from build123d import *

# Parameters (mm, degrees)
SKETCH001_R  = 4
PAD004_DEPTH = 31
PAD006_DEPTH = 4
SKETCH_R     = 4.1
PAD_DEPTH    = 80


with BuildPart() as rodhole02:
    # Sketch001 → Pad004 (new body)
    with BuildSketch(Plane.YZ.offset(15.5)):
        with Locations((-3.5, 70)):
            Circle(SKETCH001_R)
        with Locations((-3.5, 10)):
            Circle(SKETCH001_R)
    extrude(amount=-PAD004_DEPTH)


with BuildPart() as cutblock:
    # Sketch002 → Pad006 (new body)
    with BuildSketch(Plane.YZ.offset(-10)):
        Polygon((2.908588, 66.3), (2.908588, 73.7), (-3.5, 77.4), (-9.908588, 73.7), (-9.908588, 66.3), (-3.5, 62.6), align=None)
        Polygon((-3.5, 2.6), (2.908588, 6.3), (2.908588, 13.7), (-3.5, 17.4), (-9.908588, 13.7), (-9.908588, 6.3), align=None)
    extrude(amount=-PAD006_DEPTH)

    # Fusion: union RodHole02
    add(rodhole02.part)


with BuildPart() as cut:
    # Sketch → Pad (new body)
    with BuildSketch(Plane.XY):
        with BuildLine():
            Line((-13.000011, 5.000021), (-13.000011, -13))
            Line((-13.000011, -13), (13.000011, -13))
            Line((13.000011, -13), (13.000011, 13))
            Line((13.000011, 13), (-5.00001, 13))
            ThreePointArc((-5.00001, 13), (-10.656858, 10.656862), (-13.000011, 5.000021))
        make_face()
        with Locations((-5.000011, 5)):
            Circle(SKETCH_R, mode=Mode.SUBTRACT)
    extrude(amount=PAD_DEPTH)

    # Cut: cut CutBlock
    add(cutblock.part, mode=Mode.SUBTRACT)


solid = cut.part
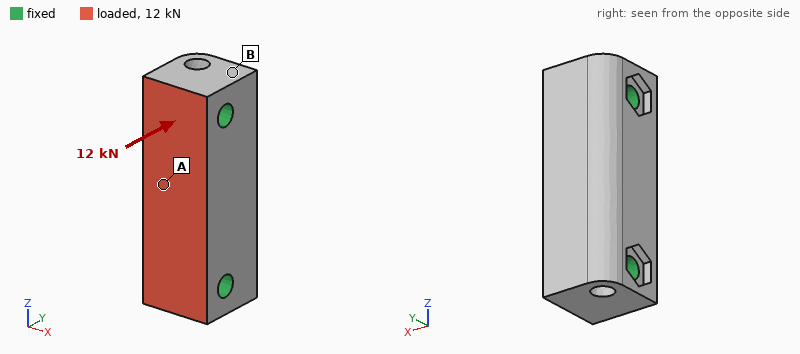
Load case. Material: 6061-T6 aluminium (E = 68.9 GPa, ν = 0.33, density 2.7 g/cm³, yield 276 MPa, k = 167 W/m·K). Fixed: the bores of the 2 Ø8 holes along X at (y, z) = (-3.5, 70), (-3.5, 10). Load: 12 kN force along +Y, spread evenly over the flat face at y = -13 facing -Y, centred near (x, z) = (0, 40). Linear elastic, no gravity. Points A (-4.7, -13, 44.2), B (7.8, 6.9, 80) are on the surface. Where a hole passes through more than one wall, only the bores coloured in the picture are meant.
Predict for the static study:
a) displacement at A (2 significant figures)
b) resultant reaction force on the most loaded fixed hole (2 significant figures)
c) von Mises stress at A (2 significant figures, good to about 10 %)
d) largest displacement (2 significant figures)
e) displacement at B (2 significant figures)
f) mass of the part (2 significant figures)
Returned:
9.6 µm
6.0 kN
12 MPa
11 µm
1.9 µm
120 g
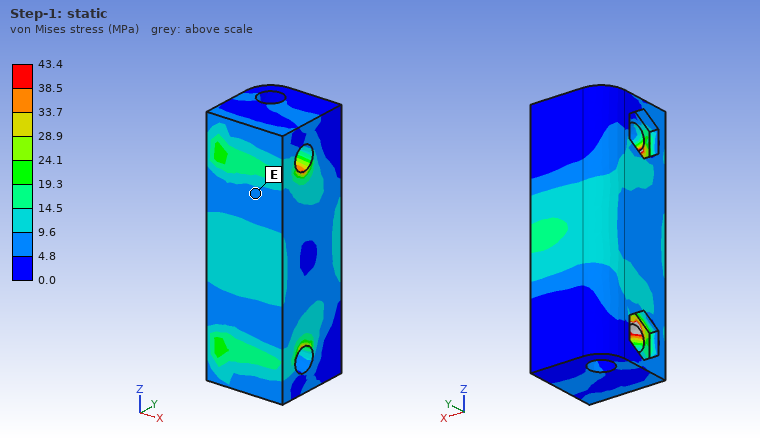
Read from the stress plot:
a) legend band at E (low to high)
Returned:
4.8 to 9.6 MPa
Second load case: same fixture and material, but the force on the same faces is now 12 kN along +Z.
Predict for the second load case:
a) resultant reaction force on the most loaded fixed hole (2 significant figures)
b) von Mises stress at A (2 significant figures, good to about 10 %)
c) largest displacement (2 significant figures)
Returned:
6.2 kN
10 MPa
5.1 µm
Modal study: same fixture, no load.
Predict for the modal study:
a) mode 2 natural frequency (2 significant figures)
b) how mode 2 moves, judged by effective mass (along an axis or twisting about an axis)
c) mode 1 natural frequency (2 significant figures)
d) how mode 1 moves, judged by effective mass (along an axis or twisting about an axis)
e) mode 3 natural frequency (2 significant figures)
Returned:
18 kHz
along X
17 kHz
along Y
22 kHz
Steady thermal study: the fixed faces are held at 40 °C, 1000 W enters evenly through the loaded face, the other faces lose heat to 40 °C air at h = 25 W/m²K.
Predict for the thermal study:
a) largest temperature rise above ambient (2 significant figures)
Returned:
80 K
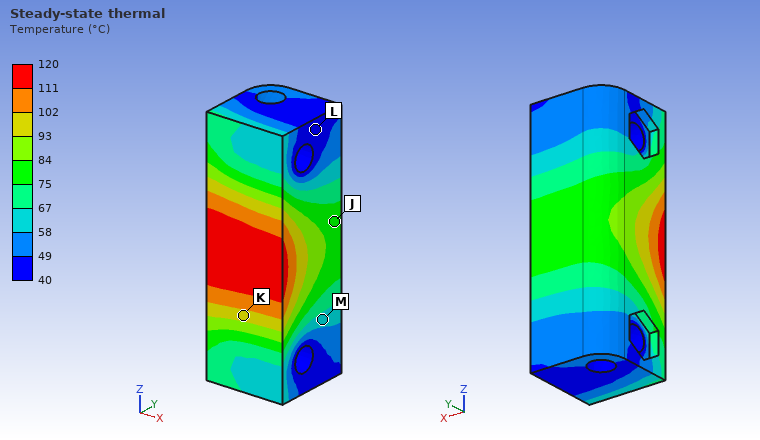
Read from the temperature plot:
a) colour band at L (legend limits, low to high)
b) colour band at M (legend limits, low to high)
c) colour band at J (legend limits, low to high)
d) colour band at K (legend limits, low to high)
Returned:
40 to 49 °C
58 to 67 °C
75 to 84 °C
93 to 102 °C
